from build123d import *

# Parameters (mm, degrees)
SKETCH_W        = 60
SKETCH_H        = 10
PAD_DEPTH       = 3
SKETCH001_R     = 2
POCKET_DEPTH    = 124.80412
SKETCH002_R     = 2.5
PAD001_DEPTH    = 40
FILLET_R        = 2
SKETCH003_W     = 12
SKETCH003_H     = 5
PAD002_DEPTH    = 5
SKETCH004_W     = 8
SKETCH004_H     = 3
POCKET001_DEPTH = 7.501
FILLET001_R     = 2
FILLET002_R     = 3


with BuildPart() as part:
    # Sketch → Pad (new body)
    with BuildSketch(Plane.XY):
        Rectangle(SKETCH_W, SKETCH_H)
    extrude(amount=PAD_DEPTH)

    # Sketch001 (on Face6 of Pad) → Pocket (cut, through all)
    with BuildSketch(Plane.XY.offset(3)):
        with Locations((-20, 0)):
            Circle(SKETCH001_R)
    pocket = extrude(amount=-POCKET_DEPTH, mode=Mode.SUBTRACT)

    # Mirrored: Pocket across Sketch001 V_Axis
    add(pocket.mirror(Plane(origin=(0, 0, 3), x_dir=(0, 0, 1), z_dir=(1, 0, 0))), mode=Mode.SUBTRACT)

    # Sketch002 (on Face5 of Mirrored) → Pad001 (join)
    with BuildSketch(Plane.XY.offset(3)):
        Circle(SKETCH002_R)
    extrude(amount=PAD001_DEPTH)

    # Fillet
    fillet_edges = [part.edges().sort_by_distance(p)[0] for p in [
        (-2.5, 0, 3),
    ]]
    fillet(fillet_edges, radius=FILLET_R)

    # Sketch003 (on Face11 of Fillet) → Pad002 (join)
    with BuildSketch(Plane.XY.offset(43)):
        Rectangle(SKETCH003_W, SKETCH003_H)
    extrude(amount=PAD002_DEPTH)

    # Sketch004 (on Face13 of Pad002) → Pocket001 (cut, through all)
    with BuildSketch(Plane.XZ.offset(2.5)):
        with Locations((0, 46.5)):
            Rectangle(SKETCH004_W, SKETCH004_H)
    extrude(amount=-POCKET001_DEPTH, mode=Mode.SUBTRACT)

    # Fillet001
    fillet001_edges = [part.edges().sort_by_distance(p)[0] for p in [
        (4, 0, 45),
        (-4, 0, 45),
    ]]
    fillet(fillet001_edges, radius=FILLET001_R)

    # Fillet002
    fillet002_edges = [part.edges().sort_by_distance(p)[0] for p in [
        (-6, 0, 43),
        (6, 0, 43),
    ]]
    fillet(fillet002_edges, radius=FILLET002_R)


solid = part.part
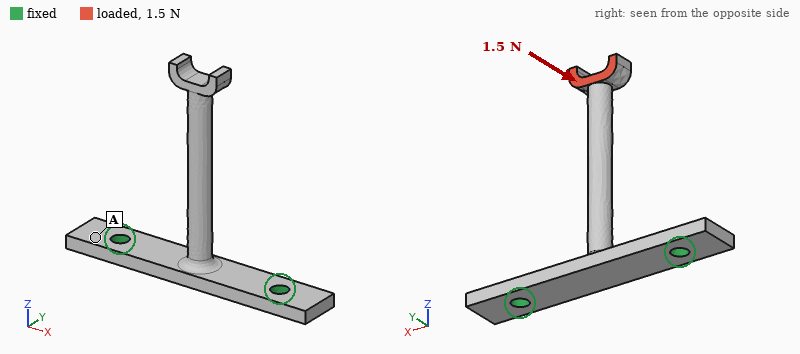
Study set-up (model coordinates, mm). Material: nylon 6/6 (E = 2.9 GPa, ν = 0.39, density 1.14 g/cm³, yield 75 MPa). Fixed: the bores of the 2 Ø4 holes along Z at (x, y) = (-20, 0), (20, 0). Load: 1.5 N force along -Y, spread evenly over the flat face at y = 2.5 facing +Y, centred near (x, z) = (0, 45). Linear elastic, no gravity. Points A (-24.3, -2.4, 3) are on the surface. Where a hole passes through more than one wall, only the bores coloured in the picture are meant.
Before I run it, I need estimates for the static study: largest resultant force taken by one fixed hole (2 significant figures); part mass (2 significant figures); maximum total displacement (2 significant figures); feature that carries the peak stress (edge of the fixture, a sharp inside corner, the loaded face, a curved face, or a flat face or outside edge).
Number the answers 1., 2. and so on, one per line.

1. 0.75 N
2. 3.1 g
3. 0.75 mm
4. a curved face
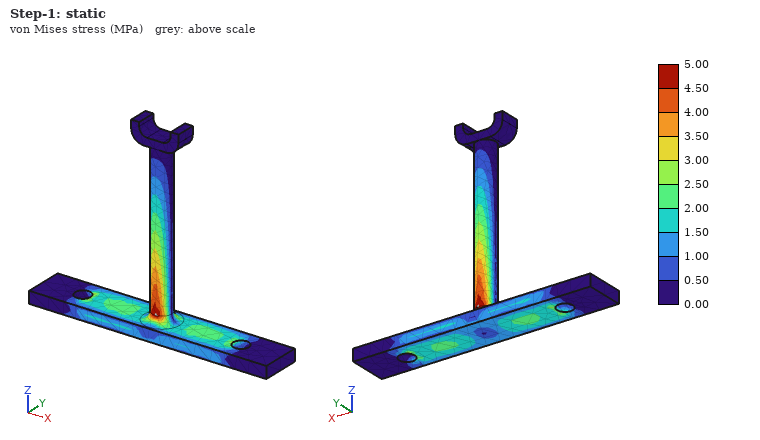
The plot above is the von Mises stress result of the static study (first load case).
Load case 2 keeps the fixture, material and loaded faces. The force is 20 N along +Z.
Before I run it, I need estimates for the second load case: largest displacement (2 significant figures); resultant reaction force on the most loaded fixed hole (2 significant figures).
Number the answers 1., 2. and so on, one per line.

1. 0.81 mm
2. 10 N
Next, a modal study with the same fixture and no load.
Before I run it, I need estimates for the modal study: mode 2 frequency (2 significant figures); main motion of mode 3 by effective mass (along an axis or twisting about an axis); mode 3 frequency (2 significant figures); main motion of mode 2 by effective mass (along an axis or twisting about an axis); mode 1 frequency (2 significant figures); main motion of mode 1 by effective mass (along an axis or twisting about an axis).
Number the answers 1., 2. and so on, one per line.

1. 450 Hz
2. along Z
3. 2100 Hz
4. along X
5. 370 Hz
6. along Y
